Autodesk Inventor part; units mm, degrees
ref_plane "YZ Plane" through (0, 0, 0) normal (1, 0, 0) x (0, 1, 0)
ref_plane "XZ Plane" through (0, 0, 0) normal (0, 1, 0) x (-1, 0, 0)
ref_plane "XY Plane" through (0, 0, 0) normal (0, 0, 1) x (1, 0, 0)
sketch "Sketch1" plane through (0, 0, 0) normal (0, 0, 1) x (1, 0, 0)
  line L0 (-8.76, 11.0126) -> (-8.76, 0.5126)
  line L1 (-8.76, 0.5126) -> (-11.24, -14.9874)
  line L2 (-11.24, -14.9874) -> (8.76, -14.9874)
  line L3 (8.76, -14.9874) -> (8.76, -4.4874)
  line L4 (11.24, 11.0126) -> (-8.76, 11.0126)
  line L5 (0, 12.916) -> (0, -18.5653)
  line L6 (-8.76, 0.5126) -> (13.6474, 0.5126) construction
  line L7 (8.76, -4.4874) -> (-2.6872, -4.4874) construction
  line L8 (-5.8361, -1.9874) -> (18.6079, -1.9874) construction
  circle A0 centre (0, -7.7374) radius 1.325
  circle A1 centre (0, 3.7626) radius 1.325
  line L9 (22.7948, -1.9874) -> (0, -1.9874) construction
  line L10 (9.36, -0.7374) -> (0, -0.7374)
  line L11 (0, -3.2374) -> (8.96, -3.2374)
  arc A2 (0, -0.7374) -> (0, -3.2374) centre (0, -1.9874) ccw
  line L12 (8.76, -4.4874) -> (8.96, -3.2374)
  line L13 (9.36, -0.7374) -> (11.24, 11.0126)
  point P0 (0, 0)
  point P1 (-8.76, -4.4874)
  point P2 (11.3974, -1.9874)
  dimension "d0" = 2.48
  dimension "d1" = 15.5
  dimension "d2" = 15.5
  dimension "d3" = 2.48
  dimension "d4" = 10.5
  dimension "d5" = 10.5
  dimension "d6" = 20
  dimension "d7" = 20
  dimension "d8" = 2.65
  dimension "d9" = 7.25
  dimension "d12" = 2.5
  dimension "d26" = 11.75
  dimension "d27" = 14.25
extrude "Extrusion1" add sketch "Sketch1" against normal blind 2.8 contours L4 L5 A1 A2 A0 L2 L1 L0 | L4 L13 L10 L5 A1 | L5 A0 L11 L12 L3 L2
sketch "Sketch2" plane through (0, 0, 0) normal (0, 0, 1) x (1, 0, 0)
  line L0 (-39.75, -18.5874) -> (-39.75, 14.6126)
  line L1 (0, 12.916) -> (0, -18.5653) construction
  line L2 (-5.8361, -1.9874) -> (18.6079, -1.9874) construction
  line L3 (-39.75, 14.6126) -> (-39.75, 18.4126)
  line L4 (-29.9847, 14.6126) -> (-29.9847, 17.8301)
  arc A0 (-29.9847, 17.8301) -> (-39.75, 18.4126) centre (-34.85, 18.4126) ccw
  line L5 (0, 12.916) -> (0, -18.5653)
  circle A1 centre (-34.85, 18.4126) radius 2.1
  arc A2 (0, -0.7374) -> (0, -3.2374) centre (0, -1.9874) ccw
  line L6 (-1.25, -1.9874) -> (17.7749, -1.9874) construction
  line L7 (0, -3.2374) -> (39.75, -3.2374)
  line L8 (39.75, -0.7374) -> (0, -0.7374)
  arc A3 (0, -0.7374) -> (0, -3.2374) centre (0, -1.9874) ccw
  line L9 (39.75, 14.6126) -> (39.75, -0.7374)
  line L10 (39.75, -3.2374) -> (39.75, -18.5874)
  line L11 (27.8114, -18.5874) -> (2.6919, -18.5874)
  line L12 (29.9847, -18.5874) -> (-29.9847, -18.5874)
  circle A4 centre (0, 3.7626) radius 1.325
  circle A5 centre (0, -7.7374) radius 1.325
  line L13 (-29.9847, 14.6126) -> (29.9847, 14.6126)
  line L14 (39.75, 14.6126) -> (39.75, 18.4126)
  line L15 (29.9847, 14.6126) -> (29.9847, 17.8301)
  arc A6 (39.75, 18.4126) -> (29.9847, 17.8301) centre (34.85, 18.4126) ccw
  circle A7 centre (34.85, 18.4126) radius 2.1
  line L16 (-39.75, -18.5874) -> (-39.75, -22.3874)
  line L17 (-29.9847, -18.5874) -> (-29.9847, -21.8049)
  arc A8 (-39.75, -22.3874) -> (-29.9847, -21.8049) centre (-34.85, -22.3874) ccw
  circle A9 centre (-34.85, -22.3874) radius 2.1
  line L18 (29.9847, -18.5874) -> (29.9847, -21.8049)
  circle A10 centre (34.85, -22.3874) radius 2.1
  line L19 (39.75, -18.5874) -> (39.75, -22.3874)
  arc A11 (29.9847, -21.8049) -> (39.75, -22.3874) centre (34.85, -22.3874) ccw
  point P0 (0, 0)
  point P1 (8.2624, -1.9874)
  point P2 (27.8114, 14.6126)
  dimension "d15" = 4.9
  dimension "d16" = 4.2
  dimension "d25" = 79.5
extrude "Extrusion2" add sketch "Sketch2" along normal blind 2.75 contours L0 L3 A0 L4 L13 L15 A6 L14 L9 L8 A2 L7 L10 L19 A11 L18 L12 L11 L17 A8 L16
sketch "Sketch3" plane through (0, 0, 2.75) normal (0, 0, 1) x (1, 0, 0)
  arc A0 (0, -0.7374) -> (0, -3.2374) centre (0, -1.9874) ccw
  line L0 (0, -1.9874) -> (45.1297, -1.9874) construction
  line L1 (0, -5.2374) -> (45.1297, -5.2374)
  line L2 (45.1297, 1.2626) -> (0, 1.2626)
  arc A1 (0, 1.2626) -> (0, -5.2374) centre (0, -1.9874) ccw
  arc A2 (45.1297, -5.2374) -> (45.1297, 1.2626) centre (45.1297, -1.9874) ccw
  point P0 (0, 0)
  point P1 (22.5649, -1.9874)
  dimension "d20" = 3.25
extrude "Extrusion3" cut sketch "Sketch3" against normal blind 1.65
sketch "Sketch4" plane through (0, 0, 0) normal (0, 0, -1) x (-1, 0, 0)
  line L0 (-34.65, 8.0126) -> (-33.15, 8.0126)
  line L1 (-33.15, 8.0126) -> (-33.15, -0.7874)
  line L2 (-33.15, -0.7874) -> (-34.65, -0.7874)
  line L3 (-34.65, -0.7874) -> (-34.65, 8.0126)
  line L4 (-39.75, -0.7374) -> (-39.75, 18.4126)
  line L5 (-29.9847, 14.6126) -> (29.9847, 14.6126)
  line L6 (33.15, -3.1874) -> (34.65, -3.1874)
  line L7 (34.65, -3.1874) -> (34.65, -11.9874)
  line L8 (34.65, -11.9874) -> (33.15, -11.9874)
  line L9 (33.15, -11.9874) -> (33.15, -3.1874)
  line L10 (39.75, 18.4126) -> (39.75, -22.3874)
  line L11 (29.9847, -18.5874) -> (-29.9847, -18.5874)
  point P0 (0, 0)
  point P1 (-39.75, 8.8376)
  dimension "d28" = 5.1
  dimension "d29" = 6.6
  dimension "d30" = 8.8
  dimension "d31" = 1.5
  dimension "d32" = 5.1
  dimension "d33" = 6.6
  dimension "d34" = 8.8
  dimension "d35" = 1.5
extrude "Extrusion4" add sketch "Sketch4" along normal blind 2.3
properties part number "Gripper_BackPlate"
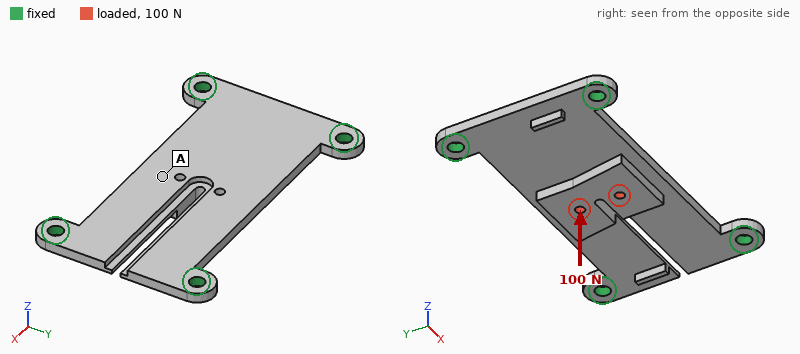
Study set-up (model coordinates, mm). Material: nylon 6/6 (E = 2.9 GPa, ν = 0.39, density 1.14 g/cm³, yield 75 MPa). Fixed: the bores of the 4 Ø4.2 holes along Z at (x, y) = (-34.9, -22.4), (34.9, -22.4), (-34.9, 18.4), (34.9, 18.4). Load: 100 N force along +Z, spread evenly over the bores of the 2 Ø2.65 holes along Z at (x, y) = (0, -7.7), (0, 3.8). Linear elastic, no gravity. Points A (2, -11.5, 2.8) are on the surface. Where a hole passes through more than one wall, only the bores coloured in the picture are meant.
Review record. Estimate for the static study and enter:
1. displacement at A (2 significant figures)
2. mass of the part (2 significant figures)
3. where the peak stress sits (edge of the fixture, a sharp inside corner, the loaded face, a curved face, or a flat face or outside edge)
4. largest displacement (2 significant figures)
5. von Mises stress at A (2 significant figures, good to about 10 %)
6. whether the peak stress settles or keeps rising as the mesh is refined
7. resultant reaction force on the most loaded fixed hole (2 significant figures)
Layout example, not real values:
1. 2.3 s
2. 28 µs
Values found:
1. 0.92 mm
2. 9.9 g
3. edge of the fixture
4. 0.96 mm
5. 8.7 MPa
6. keeps rising
7. 37 N
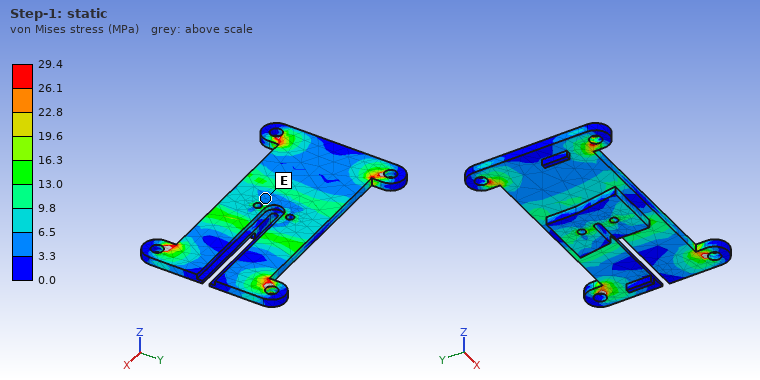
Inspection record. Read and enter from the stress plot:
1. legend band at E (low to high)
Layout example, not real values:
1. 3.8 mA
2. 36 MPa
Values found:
1. 3.3 to 6.5 MPa
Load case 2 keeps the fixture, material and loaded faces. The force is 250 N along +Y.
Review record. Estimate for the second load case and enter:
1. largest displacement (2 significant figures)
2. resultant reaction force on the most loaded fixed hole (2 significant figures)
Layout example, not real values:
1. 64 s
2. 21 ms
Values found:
1. 0.39 mm
2. 140 N
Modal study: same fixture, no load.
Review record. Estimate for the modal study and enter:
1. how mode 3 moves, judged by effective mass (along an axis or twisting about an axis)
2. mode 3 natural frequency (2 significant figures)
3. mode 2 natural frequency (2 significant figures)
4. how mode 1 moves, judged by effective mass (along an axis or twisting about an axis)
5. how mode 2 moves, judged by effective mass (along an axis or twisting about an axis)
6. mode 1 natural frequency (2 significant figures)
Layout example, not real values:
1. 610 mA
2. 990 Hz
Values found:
1. twisting about Y
2. 1900 Hz
3. 1300 Hz
4. along Z
5. twisting about X
6. 750 Hz
